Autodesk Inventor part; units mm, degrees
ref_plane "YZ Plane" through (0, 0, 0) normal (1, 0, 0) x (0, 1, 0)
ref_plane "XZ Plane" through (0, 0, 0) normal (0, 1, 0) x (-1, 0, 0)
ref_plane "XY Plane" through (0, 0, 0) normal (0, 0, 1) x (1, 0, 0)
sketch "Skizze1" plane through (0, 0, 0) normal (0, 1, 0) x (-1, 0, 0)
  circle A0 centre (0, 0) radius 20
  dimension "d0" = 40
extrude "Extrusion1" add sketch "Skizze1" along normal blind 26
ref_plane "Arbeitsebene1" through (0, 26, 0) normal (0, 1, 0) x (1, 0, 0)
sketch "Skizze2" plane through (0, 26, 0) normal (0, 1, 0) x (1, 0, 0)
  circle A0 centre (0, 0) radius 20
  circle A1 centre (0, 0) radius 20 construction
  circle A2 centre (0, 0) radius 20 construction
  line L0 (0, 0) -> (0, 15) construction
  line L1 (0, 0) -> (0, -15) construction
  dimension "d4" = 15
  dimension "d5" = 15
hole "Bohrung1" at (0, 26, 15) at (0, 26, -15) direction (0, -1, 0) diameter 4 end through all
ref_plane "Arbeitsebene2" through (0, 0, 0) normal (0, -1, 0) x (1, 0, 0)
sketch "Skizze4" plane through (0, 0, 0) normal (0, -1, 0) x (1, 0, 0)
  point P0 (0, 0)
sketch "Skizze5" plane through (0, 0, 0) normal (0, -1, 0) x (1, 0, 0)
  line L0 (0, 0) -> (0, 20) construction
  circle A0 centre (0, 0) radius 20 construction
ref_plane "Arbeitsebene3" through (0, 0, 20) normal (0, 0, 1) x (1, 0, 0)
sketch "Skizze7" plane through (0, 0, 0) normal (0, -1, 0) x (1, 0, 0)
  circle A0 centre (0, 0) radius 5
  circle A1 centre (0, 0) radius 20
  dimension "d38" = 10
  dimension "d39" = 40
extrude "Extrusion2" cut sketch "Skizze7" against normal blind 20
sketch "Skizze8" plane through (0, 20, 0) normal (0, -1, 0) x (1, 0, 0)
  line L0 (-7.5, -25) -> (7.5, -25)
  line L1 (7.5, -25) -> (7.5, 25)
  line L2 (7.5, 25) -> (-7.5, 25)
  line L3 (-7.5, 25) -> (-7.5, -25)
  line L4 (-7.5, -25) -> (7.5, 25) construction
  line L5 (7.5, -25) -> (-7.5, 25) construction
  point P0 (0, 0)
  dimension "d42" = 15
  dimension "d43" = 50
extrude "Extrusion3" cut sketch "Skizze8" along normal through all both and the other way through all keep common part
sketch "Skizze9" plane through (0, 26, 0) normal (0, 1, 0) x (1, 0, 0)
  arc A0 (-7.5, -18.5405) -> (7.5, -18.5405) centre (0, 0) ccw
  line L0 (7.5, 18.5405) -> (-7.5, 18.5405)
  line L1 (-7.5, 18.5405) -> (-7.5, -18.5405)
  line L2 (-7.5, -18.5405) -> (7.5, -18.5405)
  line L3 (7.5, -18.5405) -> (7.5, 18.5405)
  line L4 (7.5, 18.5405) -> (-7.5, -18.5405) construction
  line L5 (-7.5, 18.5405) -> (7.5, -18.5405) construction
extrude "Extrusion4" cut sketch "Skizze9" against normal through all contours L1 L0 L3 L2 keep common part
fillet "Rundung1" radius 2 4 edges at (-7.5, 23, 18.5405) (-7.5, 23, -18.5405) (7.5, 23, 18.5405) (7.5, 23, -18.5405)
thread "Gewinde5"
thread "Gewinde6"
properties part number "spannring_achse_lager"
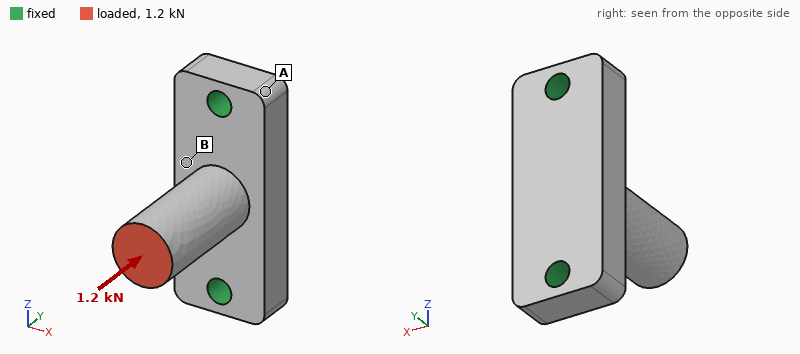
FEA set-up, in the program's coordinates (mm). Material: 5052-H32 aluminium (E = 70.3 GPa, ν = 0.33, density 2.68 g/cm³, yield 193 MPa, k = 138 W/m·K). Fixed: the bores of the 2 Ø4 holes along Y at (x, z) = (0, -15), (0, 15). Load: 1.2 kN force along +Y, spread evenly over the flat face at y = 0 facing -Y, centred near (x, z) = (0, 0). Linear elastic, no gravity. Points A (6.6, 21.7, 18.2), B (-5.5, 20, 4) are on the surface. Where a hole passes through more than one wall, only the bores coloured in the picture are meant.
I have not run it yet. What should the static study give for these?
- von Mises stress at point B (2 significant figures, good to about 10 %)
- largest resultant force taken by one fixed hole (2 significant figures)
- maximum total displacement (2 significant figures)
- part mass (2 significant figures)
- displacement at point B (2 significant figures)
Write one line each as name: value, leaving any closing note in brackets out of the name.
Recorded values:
von Mises stress at point B: 21 MPa
largest resultant force taken by one fixed hole: 610 N
maximum total displacement: 14 µm
part mass: 13 g
displacement at point B: 8.6 µm
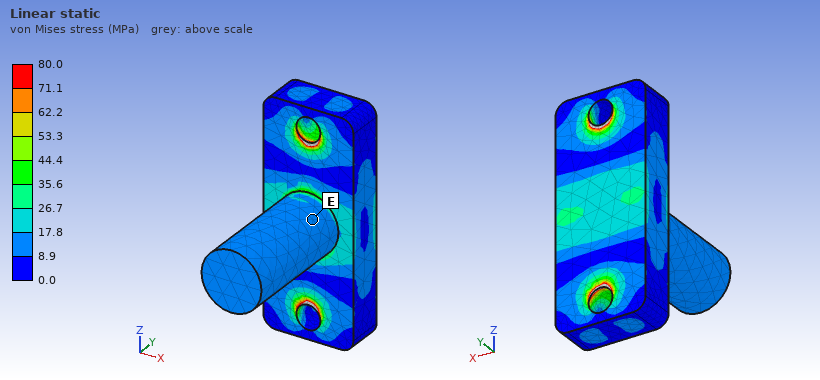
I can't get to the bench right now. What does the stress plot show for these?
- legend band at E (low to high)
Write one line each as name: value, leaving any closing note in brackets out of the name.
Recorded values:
legend band at E: 8.9 to 17.8 MPa
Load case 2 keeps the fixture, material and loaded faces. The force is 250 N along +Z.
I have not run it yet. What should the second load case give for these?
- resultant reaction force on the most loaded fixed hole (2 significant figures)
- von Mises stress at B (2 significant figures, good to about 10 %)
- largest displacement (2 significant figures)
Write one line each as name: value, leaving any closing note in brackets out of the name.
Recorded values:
resultant reaction force on the most loaded fixed hole: 290 N
von Mises stress at B: 12 MPa
largest displacement: 37 µm
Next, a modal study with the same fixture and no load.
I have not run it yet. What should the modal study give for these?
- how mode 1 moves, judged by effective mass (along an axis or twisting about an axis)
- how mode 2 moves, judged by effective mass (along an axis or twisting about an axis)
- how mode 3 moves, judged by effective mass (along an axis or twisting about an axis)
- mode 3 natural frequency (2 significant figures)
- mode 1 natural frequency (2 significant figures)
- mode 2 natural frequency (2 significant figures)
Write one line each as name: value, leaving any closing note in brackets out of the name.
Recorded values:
how mode 1 moves, judged by effective mass: along X
how mode 2 moves, judged by effective mass: along Z
how mode 3 moves, judged by effective mass: along Y
mode 3 natural frequency: 20 kHz
mode 1 natural frequency: 8300 Hz
mode 2 natural frequency: 12 kHz
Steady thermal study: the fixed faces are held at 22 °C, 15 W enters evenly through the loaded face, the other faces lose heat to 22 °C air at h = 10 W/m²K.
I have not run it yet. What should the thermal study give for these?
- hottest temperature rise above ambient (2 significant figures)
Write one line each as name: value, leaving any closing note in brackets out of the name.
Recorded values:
hottest temperature rise above ambient: 37 K
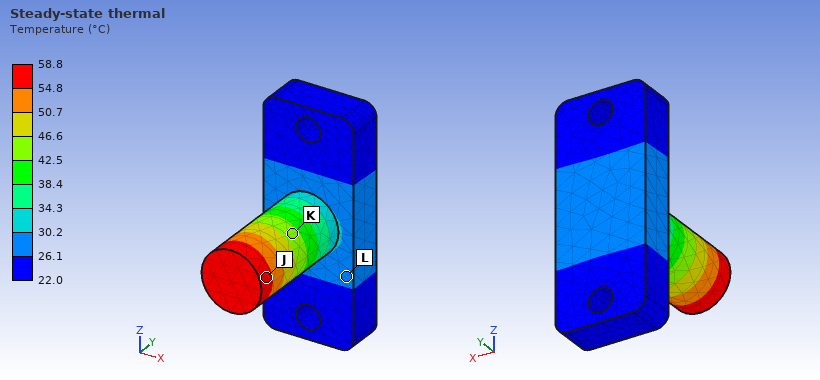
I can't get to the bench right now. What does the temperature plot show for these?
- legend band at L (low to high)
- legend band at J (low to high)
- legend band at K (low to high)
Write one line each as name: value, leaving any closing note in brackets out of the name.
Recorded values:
legend band at L: 26.1 to 30.2 °C
legend band at J: 54.8 to 58.8 °C
legend band at K: 42.5 to 46.6 °C
